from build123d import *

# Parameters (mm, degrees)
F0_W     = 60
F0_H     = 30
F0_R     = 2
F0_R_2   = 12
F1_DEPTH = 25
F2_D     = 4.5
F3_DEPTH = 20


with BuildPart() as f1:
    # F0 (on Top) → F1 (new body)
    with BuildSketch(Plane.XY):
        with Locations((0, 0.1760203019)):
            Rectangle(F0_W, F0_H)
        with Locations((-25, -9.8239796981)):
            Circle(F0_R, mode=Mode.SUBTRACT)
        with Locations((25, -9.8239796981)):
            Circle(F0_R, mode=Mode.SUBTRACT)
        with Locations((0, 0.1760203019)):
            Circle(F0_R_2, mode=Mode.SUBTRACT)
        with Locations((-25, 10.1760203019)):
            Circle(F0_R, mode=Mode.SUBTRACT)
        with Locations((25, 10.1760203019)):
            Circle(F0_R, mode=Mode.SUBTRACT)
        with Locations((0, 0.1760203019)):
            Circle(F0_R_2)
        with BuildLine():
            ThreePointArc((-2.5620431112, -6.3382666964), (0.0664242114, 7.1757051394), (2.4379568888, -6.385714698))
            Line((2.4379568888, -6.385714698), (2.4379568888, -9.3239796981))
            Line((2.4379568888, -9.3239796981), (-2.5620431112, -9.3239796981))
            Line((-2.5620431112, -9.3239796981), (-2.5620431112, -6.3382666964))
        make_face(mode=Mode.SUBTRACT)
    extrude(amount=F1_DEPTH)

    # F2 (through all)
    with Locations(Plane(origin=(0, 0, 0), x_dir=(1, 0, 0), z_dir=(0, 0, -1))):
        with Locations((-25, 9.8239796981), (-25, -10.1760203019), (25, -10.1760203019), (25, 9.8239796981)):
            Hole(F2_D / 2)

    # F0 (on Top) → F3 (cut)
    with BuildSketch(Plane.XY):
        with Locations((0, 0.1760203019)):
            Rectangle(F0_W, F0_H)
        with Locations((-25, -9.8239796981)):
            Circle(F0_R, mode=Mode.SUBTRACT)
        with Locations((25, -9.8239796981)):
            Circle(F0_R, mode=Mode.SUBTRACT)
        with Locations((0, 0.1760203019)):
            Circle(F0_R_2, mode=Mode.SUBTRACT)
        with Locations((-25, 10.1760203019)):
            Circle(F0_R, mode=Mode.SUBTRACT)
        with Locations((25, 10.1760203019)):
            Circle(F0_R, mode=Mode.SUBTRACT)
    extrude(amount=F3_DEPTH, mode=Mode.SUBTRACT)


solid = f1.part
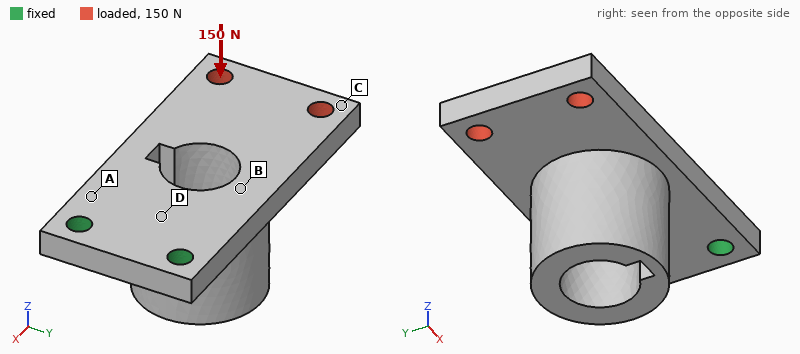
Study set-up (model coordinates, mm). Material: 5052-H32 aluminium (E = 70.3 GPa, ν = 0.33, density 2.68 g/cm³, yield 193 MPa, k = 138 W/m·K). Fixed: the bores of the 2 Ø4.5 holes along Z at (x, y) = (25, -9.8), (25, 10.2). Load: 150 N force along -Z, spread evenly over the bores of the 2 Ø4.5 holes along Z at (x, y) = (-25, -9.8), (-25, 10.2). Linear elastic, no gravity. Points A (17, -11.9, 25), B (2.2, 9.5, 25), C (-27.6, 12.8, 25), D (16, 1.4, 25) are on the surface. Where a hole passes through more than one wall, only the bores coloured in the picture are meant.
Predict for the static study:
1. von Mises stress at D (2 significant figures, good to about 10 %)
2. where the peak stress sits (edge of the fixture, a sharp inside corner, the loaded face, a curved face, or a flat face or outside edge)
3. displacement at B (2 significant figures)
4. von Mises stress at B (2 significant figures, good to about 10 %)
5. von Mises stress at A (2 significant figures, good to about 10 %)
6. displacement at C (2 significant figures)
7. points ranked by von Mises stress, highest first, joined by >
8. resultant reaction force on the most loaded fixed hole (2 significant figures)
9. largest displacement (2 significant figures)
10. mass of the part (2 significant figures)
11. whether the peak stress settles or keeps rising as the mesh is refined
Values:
40 MPa
edge of the fixture
0.070 mm
12 MPa
52 MPa
0.23 mm
A > D > B > C
85 N
0.25 mm
36 g
keeps rising
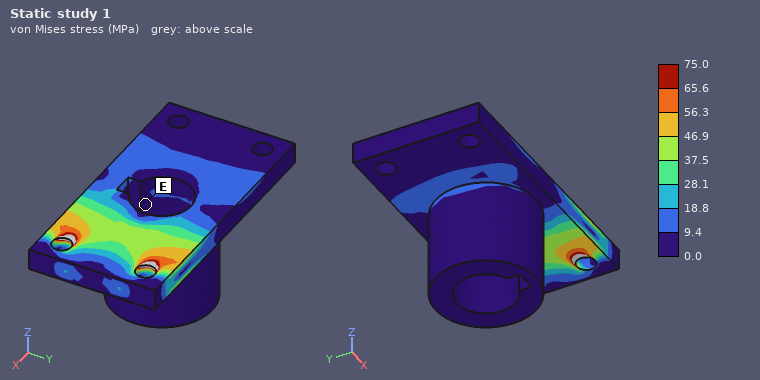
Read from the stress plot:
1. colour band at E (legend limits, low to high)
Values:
0.0 to 9.4 MPa
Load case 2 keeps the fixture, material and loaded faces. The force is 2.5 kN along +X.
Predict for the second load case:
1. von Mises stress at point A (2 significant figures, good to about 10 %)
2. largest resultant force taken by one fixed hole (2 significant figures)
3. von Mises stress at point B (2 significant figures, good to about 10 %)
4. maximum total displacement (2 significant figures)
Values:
25 MPa
1.3 kN
36 MPa
37 µm
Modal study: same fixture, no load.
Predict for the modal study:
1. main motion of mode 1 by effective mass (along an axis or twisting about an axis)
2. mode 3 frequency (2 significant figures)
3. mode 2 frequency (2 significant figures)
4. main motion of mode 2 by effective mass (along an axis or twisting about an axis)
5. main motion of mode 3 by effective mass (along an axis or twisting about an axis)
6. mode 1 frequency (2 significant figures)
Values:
along Z
5800 Hz
4100 Hz
along Y
along Y
1300 Hz
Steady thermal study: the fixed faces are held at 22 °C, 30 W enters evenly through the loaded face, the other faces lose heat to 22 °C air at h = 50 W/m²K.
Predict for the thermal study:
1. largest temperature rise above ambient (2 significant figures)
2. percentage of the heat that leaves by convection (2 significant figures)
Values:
63 K
30 %
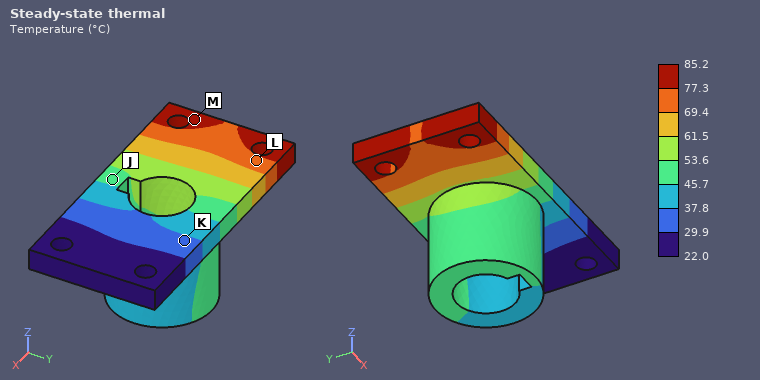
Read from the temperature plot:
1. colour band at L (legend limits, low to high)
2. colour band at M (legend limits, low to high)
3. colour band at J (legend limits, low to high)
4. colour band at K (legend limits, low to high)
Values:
69.4 to 77.3 °C
77.3 to 85.2 °C
45.7 to 53.6 °C
29.9 to 37.8 °C
